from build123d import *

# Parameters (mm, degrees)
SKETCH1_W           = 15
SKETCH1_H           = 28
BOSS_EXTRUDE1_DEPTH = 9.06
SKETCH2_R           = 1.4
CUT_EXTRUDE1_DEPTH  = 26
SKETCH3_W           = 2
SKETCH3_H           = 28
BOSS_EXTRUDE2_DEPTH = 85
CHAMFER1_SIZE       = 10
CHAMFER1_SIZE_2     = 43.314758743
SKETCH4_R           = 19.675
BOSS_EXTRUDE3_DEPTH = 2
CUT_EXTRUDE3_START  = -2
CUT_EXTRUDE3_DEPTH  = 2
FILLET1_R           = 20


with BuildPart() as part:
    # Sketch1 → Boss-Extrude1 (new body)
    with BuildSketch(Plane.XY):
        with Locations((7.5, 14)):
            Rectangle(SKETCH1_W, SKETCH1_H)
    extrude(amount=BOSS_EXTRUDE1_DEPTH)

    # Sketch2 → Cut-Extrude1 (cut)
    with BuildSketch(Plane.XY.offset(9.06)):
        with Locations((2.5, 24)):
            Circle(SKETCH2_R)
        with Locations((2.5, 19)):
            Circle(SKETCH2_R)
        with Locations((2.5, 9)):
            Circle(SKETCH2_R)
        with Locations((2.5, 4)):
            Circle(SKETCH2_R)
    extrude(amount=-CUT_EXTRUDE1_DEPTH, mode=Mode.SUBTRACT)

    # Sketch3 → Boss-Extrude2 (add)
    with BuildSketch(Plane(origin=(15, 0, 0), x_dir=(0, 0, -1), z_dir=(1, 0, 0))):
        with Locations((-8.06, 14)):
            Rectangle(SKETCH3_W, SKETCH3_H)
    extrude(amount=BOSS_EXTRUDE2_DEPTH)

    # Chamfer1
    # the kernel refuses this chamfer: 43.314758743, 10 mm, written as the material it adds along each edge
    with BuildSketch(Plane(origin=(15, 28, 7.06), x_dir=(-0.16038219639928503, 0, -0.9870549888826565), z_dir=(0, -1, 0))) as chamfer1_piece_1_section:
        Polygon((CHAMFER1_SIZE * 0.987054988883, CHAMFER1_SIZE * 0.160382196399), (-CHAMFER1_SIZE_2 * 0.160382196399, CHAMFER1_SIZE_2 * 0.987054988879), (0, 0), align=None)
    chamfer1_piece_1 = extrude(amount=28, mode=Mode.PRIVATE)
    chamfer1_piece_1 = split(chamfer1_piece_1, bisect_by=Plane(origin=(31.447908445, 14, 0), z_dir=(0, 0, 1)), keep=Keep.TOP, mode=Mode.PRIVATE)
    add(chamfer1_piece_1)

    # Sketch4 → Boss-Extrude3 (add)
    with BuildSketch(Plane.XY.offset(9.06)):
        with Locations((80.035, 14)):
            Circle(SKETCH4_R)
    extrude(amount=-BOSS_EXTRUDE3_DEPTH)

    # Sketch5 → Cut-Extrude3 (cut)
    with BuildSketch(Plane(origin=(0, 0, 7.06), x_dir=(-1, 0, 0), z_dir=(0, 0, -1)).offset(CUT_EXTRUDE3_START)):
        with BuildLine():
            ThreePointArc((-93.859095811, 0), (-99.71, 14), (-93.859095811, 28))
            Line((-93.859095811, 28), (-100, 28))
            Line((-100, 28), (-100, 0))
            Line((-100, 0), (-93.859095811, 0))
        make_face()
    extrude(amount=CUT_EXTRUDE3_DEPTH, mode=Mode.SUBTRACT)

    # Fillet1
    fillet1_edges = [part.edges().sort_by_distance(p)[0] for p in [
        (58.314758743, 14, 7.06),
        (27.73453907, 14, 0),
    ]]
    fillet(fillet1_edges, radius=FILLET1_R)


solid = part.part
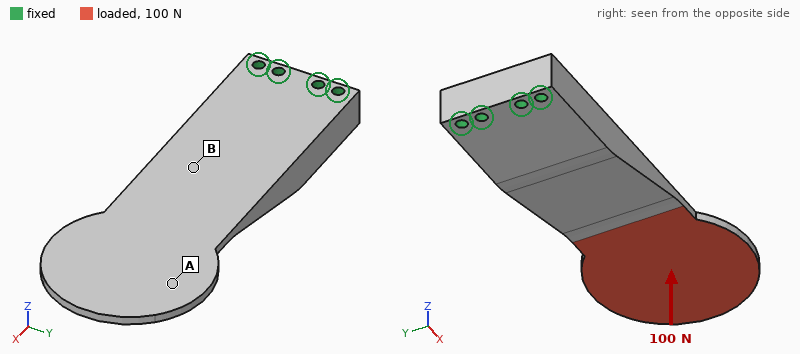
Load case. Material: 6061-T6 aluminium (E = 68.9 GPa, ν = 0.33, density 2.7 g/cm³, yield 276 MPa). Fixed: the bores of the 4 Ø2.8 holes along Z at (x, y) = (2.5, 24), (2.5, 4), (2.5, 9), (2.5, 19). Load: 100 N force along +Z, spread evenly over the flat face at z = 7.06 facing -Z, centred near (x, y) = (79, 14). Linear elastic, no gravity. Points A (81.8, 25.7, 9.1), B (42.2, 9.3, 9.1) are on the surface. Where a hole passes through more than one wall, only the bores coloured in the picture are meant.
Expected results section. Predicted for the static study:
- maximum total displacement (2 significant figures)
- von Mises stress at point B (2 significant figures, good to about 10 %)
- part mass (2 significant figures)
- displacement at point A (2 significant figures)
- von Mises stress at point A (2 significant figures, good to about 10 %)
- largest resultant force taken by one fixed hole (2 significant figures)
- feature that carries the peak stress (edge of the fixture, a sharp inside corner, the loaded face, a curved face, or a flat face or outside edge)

1.1 mm
26 MPa
38 g
0.61 mm
12 MPa
65 N
a flat face or outside edge
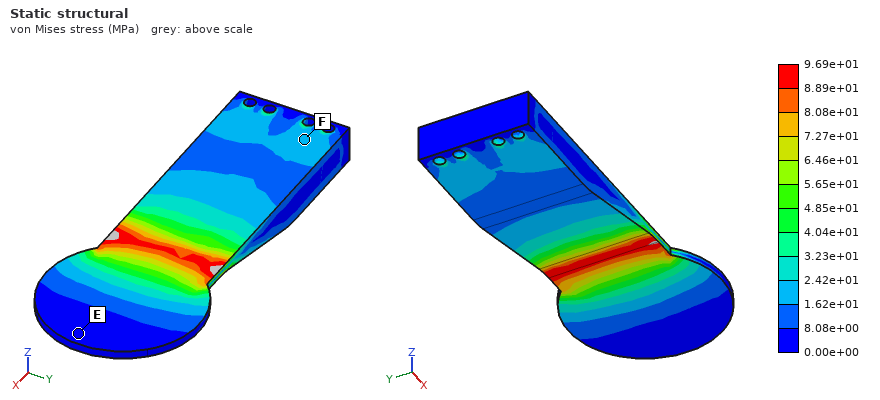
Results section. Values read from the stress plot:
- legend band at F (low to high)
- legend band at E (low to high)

1.62e+01 to 2.42e+01 MPa
0.00e+00 to 8.08e+00 MPa
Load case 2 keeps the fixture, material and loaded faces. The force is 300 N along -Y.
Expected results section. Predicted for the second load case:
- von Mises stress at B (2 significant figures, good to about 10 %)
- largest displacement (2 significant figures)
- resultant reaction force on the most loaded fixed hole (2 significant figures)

7.8 MPa
0.11 mm
920 N
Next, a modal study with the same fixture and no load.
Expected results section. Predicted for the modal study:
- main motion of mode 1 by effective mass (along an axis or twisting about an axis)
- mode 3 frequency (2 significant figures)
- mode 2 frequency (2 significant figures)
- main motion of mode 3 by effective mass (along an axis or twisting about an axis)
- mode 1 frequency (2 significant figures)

along Z
2800 Hz
2200 Hz
along Z
730 Hz
